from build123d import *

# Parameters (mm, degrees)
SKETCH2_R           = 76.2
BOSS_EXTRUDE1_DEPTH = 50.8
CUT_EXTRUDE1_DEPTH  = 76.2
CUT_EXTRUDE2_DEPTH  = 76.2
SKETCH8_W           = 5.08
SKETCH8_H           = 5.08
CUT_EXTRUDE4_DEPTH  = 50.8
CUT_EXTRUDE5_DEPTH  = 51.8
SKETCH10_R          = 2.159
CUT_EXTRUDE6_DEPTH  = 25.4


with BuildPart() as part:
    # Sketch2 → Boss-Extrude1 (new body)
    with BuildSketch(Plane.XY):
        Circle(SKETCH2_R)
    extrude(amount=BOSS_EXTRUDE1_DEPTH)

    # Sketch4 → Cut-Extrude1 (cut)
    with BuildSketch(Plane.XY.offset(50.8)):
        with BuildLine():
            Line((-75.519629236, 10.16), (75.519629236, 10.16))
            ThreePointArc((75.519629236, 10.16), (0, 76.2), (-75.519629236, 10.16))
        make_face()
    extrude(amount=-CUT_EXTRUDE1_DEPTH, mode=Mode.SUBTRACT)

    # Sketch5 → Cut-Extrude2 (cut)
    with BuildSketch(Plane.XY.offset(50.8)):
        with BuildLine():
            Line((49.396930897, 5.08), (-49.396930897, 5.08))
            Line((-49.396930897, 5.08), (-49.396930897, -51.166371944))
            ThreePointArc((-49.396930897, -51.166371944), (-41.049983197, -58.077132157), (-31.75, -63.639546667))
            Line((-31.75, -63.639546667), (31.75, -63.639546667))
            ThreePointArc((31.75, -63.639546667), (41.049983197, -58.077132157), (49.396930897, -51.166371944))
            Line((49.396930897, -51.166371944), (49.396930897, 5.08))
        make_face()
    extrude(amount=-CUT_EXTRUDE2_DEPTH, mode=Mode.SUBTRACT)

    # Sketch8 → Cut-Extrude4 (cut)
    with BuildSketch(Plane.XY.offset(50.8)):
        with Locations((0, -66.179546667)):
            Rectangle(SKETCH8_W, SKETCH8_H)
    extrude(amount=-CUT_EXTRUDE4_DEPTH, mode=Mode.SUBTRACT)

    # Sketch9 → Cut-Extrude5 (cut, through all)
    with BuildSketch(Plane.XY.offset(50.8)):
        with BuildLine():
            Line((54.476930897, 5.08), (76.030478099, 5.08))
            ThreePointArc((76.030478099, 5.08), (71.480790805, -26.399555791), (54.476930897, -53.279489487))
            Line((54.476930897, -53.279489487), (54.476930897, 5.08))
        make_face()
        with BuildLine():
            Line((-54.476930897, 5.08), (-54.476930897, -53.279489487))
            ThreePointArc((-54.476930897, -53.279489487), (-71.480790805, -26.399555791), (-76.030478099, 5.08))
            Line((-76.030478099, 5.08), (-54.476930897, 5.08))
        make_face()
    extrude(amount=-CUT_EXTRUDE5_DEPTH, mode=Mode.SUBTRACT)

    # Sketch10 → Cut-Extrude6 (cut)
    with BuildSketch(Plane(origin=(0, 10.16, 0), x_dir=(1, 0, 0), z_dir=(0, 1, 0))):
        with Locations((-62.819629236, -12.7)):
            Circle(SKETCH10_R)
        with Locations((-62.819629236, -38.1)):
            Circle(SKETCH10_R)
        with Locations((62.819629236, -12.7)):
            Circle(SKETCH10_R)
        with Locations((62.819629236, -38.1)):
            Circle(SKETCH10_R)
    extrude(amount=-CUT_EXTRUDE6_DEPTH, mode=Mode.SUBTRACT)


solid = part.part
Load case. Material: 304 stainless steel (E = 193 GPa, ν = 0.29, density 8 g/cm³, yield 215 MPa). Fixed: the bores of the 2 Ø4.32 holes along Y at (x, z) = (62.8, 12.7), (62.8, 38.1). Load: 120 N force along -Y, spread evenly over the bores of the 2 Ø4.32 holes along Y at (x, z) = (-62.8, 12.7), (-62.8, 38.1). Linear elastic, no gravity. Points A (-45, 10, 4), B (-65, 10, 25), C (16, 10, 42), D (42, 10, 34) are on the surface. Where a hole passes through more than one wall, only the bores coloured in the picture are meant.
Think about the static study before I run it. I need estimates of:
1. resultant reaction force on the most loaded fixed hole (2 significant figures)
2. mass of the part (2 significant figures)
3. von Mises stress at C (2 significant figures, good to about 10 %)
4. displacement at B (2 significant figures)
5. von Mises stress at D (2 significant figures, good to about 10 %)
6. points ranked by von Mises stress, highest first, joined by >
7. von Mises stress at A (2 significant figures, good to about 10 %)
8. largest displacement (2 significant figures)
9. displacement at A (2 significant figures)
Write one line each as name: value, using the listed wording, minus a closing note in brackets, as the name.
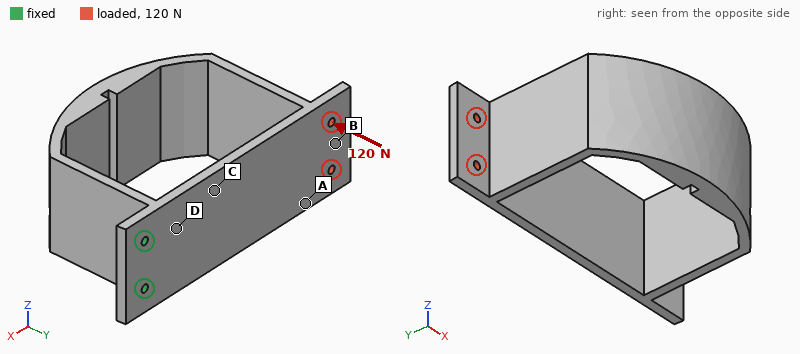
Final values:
resultant reaction force on the most loaded fixed hole: 60 N
mass of the part: 900 g
von Mises stress at C: 17 MPa
displacement at B: 0.38 mm
von Mises stress at D: 26 MPa
points ranked by von Mises stress, highest first, joined by >: D > C > A > B
von Mises stress at A: 9.9 MPa
largest displacement: 0.42 mm
displacement at A: 0.31 mm
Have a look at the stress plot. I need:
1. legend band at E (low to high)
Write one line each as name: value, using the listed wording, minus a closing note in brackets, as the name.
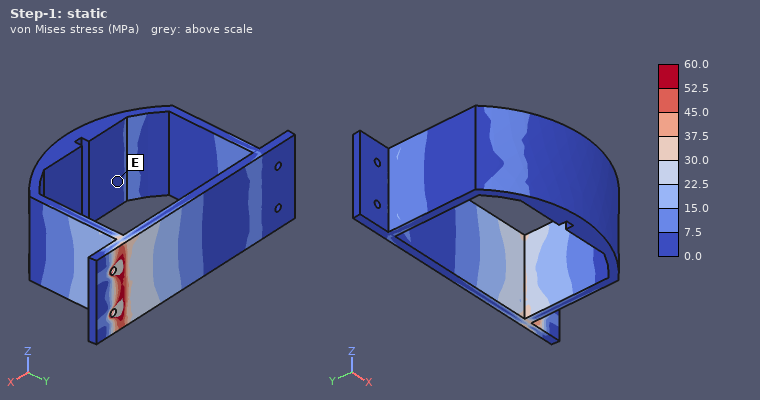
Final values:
legend band at E: 0.0 to 7.5 MPa
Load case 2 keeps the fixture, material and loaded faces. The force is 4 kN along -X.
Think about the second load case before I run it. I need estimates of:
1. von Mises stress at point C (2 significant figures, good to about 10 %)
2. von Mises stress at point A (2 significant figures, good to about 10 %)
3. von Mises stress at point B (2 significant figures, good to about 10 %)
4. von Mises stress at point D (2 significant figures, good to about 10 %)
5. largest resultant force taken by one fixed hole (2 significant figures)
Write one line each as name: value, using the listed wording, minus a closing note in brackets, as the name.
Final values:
von Mises stress at point C: 16 MPa
von Mises stress at point A: 15 MPa
von Mises stress at point B: 6.6 MPa
von Mises stress at point D: 17 MPa
largest resultant force taken by one fixed hole: 2.0 kN
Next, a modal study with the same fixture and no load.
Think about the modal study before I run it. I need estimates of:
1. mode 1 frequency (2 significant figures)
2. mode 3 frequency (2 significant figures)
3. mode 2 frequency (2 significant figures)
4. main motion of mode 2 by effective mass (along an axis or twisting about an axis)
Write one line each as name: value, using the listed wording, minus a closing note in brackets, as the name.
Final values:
mode 1 frequency: 140 Hz
mode 3 frequency: 630 Hz
mode 2 frequency: 500 Hz
main motion of mode 2 by effective mass: along Z
